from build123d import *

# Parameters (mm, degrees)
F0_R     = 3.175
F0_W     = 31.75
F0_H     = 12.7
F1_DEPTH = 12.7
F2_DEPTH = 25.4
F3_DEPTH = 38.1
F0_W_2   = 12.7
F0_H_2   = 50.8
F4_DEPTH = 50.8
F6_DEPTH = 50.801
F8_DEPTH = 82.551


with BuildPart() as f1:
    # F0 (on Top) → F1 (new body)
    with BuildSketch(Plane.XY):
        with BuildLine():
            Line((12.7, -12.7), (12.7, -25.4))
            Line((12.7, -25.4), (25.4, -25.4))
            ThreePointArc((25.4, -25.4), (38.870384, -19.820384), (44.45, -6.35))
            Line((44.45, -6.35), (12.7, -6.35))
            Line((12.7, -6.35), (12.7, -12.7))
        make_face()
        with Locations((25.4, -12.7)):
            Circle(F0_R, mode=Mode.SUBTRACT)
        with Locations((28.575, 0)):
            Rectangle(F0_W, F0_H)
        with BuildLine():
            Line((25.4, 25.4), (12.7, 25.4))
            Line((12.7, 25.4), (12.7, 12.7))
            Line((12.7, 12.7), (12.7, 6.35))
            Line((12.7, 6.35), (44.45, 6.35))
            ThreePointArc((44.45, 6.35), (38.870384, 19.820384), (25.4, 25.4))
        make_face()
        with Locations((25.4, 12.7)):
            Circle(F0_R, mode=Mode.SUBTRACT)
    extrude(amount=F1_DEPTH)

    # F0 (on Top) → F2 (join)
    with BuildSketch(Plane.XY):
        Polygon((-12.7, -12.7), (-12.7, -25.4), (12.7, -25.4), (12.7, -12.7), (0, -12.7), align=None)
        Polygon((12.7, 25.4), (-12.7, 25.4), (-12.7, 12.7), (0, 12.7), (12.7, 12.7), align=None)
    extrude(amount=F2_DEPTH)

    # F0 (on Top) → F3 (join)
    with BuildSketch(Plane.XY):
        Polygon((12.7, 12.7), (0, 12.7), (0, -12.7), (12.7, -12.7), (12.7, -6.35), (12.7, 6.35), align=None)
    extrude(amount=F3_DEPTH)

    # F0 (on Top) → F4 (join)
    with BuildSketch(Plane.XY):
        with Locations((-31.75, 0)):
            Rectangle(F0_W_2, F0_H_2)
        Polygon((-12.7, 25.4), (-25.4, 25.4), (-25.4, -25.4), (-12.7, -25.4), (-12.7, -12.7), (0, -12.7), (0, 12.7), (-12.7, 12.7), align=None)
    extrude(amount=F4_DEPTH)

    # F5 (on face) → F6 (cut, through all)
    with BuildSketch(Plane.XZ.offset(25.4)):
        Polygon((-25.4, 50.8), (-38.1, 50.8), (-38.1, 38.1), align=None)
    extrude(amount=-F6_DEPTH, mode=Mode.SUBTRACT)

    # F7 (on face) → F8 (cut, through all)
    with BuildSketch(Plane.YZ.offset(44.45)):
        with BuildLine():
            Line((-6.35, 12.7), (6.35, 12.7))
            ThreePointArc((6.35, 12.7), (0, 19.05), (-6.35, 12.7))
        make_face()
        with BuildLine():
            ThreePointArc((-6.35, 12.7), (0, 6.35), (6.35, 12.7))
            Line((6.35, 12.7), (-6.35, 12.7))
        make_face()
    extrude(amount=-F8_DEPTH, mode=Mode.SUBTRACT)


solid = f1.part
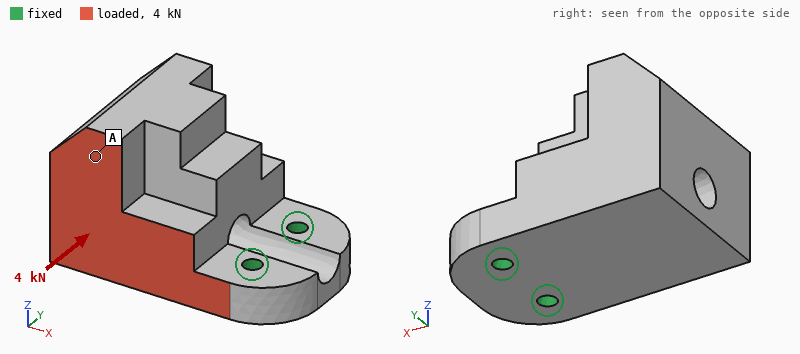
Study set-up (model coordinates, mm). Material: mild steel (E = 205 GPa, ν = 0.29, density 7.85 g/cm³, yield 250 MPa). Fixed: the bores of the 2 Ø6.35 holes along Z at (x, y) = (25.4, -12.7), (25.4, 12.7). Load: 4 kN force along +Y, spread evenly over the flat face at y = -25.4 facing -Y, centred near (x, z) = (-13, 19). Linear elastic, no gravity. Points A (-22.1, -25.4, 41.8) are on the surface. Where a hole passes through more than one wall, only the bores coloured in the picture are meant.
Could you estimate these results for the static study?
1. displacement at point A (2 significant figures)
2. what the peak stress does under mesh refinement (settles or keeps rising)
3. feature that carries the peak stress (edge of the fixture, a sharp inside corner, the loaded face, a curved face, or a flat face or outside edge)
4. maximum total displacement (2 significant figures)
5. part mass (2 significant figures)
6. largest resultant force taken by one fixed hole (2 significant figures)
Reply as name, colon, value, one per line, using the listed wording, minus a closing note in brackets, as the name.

displacement at point A: 16 µm
what the peak stress does under mesh refinement: keeps rising
feature that carries the peak stress: edge of the fixture
maximum total displacement: 18 µm
part mass: 910 g
largest resultant force taken by one fixed hole: 5.5 kN
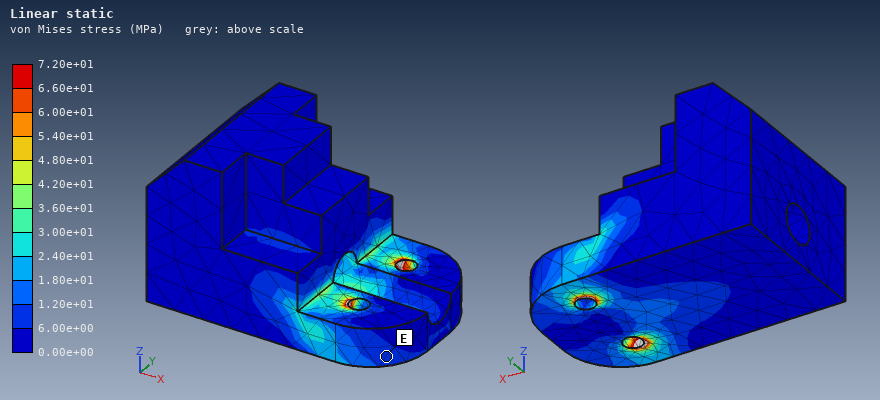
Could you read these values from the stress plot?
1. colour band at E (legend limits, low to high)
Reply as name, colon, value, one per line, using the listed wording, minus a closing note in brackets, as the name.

colour band at E: 6.00e+00 to 1.20e+01 MPa
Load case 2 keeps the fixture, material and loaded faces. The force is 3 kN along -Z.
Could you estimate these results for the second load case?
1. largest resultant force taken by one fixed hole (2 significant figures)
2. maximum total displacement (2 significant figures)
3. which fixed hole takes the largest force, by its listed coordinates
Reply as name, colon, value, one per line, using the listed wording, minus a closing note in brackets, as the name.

largest resultant force taken by one fixed hole: 3.6 kN
maximum total displacement: 81 µm
which fixed hole takes the largest force, by its listed coordinates: (25.4, -12.7)
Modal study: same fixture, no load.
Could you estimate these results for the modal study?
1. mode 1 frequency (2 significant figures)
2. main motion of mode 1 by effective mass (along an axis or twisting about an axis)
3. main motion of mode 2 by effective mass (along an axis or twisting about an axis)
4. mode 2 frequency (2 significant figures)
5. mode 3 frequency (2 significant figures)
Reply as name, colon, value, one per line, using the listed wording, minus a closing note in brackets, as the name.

mode 1 frequency: 1200 Hz
main motion of mode 1 by effective mass: along Z
main motion of mode 2 by effective mass: along Y
mode 2 frequency: 3000 Hz
mode 3 frequency: 5200 Hz
